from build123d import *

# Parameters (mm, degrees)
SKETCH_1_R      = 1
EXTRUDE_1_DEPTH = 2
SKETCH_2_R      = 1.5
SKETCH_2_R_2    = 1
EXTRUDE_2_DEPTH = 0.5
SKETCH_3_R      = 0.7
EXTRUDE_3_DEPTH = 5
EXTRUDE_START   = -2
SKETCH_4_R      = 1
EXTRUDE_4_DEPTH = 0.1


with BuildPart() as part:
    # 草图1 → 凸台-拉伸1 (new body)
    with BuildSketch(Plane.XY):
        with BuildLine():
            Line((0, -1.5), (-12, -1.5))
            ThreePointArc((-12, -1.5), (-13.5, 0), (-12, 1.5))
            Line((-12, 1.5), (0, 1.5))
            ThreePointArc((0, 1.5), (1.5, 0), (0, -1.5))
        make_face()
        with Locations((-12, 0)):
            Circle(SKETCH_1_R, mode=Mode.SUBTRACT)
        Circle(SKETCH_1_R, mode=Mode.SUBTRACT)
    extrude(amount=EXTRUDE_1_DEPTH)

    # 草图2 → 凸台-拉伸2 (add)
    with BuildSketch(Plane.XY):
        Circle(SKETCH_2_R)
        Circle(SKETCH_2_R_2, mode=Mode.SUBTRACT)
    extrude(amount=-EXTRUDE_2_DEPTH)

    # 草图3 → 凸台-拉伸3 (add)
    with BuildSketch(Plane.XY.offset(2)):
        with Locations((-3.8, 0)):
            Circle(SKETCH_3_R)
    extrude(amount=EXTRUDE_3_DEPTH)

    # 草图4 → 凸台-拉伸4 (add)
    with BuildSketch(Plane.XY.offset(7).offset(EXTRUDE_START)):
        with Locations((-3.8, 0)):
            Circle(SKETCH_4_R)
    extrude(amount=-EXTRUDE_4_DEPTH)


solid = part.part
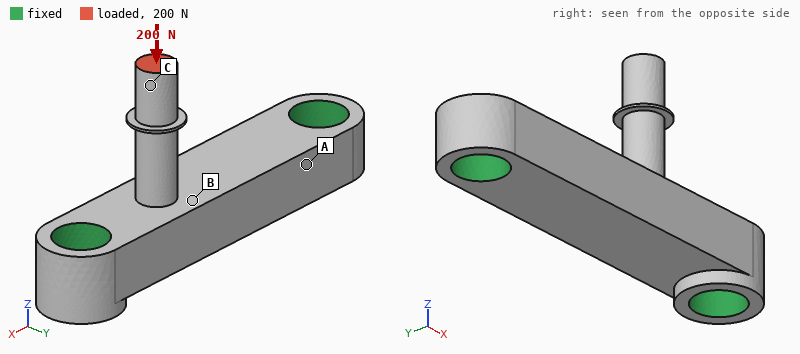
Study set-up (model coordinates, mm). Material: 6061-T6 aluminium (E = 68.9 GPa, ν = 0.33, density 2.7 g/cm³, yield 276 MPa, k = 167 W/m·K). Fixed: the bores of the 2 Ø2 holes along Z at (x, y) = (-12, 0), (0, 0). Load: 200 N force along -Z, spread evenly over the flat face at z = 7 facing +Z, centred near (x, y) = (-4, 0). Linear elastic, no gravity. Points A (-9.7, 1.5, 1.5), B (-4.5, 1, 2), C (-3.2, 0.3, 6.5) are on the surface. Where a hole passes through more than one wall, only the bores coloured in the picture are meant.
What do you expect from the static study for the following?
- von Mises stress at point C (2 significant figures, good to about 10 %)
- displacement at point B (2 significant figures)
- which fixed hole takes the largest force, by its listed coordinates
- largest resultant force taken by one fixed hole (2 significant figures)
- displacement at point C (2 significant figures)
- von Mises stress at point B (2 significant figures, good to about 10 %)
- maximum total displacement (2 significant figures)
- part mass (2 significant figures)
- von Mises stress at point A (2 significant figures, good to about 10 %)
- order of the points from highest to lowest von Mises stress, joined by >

130 MPa
7.5 µm
(0, 0)
160 N
17 µm
69 MPa
20 µm
0.23 g
19 MPa
C > B > A
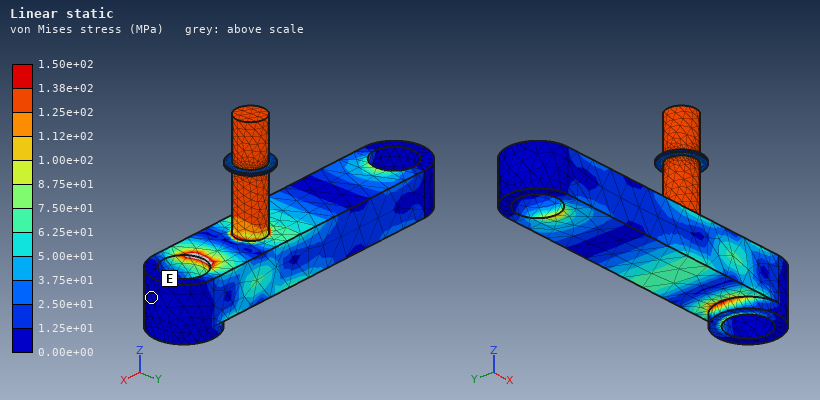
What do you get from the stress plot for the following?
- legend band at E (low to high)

0.00e+00 to 1.25e+01 MPa
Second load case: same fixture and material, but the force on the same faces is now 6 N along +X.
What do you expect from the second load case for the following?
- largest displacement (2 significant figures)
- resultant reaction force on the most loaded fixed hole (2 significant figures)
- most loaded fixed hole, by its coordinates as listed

25 µm
5.8 N
(0, 0)
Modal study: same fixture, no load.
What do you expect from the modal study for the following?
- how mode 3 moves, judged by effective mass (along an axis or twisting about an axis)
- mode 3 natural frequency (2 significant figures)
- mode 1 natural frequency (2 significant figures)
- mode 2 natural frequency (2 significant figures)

along Z
75 kHz
31 kHz
33 kHz
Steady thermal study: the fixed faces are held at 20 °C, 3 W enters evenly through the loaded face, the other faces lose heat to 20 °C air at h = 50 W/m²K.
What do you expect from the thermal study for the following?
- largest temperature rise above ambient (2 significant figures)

67 K
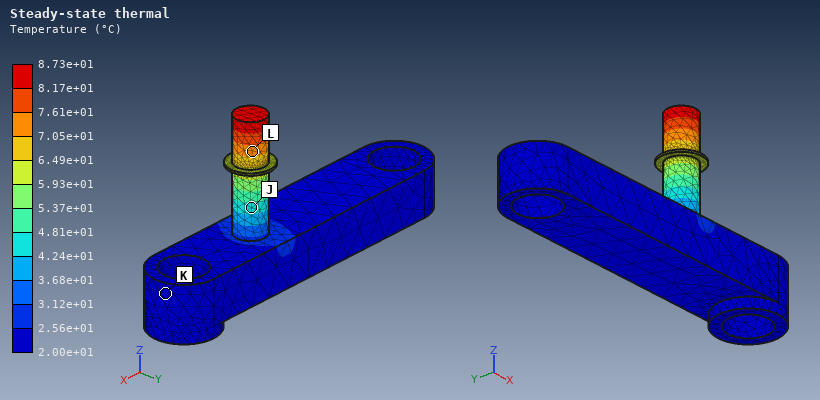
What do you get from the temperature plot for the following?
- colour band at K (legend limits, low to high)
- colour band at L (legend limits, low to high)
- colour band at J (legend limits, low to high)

2.00e+01 to 2.56e+01 °C
7.05e+01 to 7.61e+01 °C
4.24e+01 to 4.81e+01 °C
